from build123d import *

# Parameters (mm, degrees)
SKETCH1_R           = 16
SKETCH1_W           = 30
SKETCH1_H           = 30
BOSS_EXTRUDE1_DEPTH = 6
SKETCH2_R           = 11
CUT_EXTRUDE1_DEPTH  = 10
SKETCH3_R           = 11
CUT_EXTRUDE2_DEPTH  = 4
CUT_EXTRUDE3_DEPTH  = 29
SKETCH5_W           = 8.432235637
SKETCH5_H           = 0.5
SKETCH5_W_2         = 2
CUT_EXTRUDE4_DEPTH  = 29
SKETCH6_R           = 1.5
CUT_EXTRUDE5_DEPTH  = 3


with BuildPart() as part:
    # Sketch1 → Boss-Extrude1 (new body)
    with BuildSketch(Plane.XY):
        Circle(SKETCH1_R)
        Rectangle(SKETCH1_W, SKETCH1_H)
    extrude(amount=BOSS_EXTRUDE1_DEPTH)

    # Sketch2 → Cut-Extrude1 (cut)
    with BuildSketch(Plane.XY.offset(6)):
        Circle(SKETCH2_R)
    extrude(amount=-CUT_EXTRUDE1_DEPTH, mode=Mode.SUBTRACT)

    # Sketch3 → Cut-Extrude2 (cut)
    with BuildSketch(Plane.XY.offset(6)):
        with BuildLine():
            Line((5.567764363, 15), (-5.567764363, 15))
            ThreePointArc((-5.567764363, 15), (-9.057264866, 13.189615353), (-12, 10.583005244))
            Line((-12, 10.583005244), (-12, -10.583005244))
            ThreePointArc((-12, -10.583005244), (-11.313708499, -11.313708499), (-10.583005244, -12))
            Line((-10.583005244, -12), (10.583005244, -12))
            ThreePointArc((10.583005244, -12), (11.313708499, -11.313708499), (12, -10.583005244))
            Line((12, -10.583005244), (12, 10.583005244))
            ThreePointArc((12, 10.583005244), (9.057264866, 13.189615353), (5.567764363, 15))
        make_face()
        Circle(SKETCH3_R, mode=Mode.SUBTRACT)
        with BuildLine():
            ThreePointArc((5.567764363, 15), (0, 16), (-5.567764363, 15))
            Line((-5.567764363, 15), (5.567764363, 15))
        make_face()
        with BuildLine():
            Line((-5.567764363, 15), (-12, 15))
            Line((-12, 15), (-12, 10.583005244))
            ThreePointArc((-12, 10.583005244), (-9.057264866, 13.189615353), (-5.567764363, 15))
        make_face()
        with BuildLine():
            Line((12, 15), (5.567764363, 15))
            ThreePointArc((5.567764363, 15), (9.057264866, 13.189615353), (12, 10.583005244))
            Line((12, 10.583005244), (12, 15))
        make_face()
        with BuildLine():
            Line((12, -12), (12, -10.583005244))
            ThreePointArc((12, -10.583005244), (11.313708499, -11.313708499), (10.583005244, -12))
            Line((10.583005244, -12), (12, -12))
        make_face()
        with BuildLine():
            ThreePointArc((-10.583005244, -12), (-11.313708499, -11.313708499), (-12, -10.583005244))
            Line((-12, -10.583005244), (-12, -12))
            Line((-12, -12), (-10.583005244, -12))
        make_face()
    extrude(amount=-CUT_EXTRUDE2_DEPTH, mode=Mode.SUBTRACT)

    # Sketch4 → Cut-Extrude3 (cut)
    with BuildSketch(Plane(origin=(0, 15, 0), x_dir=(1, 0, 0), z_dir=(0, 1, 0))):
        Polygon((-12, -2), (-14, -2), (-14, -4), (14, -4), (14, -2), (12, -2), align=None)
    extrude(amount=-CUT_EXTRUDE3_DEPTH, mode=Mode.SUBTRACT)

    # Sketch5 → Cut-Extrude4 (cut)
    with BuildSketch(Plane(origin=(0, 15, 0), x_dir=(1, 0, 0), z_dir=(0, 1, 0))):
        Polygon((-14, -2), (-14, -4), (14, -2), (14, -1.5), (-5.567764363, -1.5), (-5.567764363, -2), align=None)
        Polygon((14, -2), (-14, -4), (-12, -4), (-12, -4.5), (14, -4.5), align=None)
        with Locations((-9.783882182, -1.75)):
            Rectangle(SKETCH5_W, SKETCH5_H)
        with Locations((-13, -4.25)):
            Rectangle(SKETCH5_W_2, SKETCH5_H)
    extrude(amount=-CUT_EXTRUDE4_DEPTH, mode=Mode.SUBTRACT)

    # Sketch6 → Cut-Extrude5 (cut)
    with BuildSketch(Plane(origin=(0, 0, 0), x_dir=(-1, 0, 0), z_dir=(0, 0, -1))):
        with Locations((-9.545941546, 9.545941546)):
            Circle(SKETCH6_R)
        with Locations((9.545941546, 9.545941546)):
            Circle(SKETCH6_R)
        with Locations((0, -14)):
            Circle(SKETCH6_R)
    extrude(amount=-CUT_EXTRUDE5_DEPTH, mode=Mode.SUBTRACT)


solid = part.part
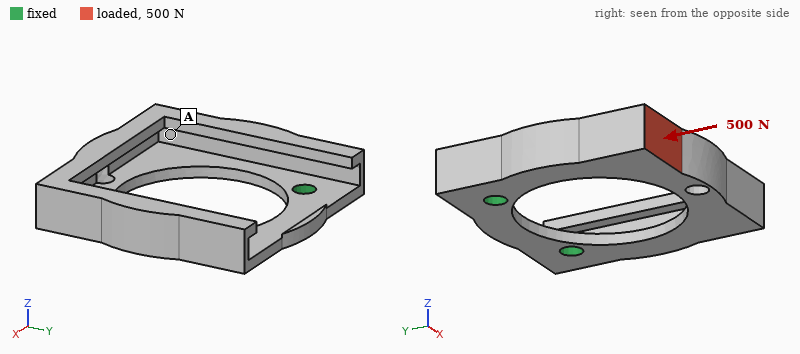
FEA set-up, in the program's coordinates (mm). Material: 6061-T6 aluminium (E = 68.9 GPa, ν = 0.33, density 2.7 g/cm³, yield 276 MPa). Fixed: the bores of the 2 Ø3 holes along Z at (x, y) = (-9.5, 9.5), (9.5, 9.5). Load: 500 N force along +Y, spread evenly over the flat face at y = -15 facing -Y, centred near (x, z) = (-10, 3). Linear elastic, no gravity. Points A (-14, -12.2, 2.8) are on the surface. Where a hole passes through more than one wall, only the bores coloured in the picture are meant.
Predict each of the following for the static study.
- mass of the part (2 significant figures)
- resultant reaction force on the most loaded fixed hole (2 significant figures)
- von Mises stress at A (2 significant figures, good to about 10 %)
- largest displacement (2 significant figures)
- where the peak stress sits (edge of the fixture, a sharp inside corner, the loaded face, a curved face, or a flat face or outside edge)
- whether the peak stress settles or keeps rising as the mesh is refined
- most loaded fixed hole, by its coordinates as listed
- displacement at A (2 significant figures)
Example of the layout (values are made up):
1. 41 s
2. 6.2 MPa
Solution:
1. 4.1 g
2. 470 N
3. 27 MPa
4. 0.25 mm
5. edge of the fixture
6. keeps rising
7. (-9.5, 9.5)
8. 0.21 mm
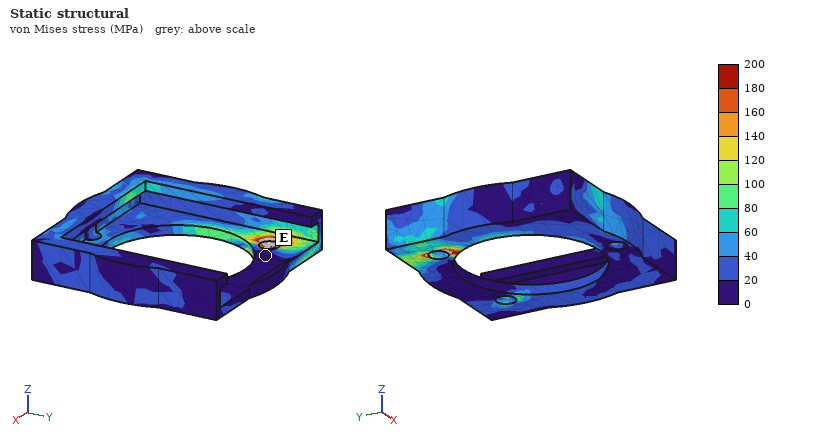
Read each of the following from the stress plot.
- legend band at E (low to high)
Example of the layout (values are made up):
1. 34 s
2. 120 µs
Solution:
1. 0 to 20 MPa
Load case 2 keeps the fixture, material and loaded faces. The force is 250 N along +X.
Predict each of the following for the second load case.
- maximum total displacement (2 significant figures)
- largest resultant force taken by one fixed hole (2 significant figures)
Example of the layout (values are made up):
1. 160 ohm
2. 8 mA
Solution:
1. 0.17 mm
2. 220 N
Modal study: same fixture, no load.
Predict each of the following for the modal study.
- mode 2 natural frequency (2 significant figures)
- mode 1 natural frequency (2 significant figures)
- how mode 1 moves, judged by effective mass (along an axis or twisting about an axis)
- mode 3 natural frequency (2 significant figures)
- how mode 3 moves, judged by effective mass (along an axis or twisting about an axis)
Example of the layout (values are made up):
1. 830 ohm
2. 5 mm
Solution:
1. 3400 Hz
2. 2100 Hz
3. along Z
4. 6500 Hz
5. along X
